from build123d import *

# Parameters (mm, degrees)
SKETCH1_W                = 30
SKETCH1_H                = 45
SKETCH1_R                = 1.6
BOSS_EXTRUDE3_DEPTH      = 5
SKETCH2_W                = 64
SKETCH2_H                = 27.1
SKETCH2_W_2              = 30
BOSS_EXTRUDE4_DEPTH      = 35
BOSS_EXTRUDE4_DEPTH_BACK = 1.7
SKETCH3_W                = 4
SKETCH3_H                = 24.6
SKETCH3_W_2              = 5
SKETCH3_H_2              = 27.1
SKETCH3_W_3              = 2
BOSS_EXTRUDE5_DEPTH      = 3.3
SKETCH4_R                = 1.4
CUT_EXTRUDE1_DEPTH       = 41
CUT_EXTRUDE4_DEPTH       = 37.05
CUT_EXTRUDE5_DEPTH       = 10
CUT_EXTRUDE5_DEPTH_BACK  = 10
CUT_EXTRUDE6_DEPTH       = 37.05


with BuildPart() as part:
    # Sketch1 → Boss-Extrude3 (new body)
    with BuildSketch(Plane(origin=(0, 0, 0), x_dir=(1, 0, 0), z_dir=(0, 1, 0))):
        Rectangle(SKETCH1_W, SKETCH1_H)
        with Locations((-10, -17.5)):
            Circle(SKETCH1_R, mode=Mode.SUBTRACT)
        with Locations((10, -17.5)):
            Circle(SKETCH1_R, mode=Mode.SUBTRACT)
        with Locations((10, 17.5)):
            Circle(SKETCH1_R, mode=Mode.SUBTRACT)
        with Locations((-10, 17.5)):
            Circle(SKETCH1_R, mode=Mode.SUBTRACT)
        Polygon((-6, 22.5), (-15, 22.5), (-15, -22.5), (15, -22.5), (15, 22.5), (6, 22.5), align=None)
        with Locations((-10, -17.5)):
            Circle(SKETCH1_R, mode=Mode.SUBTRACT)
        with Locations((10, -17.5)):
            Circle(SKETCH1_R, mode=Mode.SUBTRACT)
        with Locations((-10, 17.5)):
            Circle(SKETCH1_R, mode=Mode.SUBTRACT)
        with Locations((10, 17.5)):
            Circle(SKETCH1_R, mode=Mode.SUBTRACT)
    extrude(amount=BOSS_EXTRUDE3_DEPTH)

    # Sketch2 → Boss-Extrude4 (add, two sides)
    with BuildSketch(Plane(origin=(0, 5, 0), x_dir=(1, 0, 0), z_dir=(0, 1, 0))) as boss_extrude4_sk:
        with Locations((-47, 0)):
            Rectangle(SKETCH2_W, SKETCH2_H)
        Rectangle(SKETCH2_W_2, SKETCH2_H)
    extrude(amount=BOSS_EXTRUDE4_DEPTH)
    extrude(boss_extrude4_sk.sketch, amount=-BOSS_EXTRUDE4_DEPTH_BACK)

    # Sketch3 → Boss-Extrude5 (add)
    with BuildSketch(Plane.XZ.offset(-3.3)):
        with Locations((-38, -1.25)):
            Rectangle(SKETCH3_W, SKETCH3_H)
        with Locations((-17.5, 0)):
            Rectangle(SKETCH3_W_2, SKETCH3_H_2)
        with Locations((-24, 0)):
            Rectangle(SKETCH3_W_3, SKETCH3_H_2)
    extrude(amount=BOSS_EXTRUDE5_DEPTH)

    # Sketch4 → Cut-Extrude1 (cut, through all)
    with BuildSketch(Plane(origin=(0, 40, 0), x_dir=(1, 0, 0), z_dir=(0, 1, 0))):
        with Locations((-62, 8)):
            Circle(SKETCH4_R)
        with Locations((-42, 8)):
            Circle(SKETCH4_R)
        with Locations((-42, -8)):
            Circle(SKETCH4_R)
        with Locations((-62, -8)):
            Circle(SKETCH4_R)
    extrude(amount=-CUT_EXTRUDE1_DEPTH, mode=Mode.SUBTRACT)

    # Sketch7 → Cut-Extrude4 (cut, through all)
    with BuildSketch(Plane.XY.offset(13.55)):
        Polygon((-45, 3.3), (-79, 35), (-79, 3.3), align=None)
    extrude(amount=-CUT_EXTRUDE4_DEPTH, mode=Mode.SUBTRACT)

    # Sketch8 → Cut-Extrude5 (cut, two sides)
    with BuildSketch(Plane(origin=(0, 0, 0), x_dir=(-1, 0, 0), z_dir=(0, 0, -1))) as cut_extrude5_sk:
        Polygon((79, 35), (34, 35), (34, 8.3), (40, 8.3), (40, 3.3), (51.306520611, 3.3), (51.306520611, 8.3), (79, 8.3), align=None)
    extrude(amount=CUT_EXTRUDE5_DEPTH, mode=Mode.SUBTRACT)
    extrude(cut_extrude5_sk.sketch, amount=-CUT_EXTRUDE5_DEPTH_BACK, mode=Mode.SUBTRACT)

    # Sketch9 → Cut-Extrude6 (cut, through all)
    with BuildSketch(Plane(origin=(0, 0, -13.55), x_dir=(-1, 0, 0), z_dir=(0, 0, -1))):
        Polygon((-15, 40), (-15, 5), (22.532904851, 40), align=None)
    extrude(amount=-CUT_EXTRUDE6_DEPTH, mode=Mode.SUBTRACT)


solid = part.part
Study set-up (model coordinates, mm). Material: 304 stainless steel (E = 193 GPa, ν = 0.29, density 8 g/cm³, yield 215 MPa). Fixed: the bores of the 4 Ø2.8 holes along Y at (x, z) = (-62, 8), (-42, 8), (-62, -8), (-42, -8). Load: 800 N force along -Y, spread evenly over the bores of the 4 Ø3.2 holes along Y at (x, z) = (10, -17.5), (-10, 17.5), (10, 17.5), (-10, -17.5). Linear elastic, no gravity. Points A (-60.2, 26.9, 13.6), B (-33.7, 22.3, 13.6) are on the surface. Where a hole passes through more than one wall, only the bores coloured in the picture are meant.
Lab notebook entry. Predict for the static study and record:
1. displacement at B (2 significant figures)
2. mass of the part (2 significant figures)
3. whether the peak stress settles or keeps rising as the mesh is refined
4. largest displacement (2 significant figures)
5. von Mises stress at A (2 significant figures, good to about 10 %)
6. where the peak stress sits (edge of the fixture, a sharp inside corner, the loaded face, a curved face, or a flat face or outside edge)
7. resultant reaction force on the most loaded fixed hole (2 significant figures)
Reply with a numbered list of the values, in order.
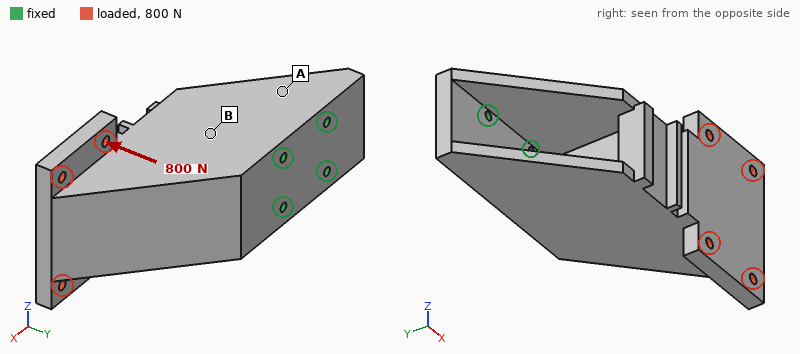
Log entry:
1. 5.1 µm
2. 400 g
3. keeps rising
4. 24 µm
5. 12 MPa
6. edge of the fixture
7. 1.1 kN
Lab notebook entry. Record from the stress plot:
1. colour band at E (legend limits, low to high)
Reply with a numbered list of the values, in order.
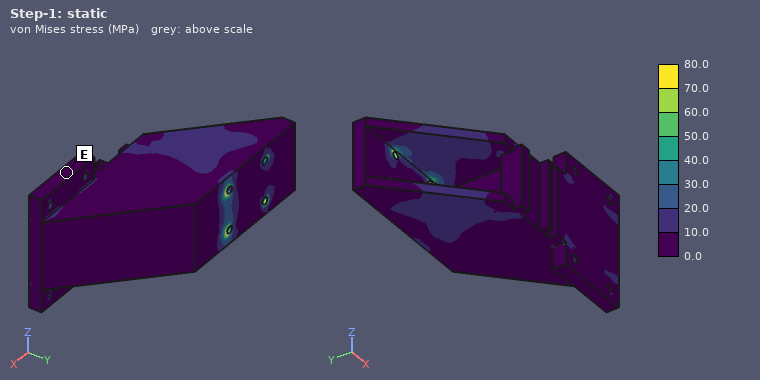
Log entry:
1. 0.0 to 10.0 MPa
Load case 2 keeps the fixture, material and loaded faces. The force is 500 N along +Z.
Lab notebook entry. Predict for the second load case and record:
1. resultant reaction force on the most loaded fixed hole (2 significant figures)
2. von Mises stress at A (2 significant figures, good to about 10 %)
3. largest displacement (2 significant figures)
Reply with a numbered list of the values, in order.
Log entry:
1. 990 N
2. 6.3 MPa
3. 13 µm
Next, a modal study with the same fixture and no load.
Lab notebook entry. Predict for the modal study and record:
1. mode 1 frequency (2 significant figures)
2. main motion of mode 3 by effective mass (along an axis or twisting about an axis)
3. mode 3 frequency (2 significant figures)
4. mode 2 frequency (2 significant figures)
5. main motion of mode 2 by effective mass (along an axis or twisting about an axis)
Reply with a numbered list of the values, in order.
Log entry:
1. 2500 Hz
2. twisting about Y
3. 5600 Hz
4. 2800 Hz
5. along Z
